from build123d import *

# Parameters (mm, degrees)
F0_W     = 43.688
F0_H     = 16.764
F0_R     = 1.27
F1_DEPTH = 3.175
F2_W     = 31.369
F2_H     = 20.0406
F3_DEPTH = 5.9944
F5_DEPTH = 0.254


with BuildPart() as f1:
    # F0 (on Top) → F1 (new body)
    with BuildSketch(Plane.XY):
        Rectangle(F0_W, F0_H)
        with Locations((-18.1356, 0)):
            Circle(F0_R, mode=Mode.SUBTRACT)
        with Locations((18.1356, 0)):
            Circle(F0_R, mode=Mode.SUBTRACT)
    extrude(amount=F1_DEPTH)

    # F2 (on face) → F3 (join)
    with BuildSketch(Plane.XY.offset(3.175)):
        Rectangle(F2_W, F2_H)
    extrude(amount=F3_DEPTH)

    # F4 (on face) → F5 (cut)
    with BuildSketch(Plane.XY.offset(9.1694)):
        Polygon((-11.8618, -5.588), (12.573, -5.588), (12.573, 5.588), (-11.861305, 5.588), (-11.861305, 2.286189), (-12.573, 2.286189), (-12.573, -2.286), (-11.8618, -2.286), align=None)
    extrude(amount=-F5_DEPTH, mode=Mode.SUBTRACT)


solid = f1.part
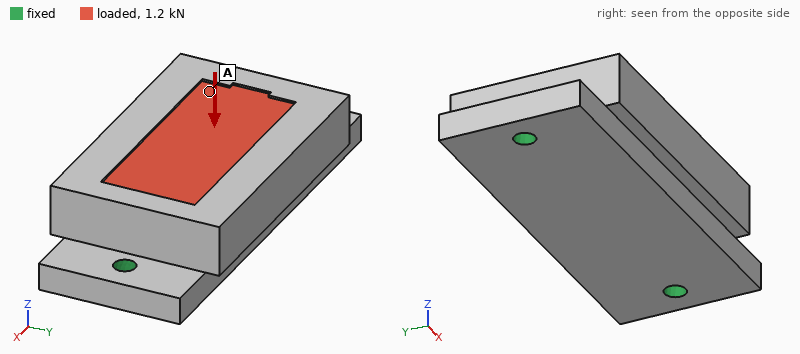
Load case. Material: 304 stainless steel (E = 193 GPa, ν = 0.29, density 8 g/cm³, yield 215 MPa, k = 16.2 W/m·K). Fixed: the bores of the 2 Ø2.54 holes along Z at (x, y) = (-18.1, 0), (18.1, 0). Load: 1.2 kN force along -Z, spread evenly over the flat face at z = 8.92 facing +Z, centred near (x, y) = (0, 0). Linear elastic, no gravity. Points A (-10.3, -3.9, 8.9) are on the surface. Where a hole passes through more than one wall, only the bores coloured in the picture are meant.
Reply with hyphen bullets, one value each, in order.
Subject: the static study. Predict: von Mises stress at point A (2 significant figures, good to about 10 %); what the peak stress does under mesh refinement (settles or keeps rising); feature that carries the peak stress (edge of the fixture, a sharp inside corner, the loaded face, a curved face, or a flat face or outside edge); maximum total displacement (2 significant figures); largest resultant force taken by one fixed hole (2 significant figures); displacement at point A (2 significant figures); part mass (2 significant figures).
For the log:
- 9.8 MPa
- keeps rising
- edge of the fixture
- 4.1 µm
- 780 N
- 3.0 µm
- 48 g
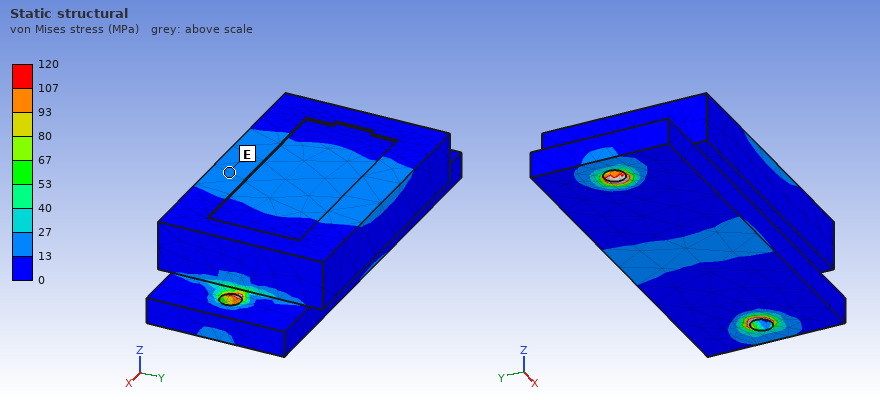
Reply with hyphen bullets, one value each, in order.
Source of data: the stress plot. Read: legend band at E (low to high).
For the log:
- 13 to 27 MPa
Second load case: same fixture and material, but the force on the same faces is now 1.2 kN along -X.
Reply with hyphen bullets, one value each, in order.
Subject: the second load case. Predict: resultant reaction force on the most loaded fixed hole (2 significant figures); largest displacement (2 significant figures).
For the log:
- 650 N
- 1.2 µm
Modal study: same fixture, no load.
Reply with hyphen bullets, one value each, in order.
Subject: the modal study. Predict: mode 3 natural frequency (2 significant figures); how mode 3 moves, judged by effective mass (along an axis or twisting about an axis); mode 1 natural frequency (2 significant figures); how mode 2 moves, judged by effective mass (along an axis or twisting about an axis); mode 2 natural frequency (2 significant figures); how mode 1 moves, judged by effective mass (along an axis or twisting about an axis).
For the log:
- 23 kHz
- along Y
- 8100 Hz
- along Z
- 15 kHz
- along Y
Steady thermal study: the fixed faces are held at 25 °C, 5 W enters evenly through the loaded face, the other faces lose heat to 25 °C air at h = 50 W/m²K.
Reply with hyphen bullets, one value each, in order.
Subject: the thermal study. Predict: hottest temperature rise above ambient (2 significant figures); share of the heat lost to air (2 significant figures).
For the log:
- 23 K
- 31 %
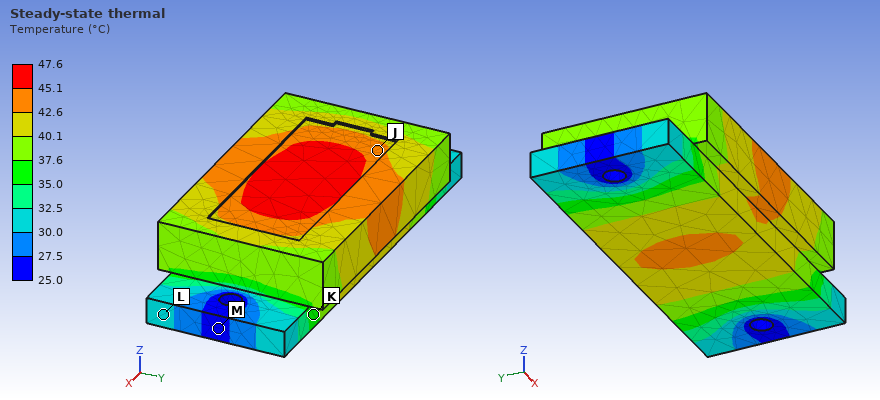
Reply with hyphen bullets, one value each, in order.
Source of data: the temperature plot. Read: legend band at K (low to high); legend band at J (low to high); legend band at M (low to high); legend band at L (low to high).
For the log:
- 35.0 to 37.6 °C
- 42.6 to 45.1 °C
- 25.0 to 27.5 °C
- 30.0 to 32.5 °C
